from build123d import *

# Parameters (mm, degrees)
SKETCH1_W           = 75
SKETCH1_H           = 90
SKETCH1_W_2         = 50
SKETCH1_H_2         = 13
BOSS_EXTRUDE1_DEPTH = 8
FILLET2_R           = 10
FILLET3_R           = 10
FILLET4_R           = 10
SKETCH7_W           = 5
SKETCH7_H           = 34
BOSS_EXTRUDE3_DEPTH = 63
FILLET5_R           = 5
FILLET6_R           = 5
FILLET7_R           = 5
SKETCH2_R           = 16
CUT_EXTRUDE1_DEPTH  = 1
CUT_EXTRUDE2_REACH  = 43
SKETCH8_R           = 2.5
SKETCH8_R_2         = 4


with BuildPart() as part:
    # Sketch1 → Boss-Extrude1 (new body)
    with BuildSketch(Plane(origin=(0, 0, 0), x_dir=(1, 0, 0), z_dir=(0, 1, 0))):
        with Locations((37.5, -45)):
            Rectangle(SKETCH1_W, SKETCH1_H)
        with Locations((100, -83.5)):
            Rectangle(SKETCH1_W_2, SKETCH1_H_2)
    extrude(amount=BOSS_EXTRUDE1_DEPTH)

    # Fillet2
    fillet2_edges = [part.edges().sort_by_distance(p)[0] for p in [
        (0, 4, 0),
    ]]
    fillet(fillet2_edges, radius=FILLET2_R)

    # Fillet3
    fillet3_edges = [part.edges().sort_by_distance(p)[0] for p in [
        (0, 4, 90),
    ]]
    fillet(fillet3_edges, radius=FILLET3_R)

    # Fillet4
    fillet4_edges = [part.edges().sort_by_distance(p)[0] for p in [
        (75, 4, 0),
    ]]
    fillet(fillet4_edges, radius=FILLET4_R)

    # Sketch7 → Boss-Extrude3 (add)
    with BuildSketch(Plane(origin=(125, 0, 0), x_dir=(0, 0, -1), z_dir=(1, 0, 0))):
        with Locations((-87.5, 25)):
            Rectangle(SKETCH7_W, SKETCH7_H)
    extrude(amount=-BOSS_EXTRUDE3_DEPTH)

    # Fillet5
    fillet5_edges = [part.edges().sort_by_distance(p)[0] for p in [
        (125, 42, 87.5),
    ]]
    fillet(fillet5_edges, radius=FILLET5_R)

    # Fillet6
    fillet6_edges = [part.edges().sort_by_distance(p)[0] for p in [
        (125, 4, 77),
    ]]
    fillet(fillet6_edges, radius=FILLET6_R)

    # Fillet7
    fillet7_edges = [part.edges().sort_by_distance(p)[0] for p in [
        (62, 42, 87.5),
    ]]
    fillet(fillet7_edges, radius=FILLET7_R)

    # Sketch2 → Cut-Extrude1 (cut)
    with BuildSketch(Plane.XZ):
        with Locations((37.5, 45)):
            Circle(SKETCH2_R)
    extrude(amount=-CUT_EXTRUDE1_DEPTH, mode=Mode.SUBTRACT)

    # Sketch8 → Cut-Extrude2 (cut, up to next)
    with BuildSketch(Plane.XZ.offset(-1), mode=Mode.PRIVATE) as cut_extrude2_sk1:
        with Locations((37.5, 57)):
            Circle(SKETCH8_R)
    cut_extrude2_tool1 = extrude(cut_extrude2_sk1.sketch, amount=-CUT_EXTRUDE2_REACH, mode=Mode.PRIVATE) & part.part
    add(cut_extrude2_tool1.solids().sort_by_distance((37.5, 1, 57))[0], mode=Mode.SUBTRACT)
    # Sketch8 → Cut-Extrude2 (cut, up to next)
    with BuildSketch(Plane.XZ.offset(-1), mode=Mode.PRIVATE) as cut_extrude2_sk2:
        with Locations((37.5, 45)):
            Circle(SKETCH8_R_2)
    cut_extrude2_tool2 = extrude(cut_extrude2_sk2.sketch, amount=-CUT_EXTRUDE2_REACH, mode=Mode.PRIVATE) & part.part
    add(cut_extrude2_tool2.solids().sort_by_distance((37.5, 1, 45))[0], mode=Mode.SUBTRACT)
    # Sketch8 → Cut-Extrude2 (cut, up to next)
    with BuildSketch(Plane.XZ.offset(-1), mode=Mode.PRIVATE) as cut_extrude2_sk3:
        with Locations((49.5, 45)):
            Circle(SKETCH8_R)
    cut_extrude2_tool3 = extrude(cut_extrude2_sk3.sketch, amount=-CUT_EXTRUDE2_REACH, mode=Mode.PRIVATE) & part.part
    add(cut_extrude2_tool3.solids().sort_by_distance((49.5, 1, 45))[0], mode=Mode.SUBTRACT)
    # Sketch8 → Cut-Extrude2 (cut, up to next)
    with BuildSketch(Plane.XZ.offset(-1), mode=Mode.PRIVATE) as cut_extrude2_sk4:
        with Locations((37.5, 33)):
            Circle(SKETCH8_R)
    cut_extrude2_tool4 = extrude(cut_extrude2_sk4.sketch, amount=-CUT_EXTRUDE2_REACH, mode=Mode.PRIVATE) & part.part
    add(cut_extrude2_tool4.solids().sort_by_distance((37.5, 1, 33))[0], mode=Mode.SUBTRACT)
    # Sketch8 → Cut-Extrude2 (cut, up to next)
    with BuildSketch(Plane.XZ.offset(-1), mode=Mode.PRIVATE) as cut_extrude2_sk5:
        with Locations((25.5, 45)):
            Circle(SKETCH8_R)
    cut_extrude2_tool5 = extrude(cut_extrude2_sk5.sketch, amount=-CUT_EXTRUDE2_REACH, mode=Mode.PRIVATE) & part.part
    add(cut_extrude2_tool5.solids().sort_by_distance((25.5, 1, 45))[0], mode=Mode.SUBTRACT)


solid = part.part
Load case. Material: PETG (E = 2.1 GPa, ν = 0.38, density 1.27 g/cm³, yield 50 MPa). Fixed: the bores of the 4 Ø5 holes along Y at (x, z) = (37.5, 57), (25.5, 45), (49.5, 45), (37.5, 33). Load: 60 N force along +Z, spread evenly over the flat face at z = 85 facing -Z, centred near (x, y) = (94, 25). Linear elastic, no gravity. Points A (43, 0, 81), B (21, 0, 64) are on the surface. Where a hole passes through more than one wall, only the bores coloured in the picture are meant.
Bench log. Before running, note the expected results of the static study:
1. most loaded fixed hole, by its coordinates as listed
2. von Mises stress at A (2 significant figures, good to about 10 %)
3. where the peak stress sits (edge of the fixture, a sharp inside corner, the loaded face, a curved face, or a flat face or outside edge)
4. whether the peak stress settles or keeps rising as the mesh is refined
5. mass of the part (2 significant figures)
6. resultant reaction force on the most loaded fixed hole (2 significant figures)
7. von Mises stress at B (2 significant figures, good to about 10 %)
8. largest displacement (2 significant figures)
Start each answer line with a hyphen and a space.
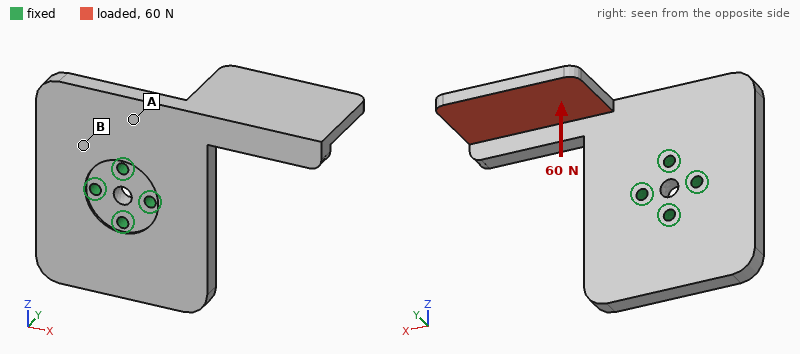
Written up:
- (49.5, 45)
- 2.2 MPa
- a sharp inside corner
- keeps rising
- 86 g
- 100 N
- 1.2 MPa
- 1.7 mm
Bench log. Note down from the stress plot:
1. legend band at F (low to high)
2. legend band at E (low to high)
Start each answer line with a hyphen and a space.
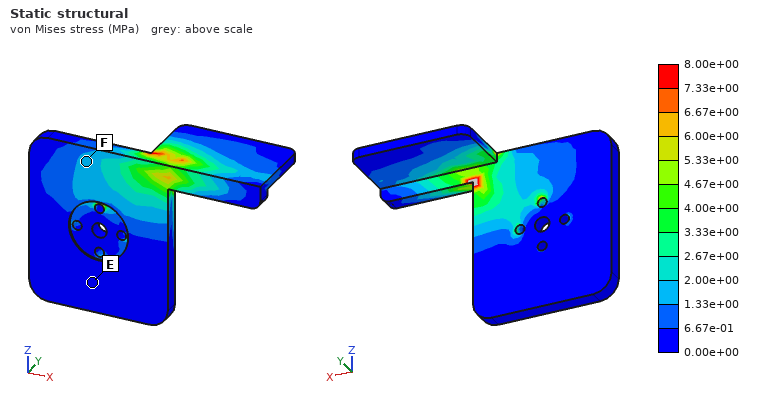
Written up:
- 1.33e+00 to 2.00e+00 MPa
- 0.00e+00 to 6.67e-01 MPa
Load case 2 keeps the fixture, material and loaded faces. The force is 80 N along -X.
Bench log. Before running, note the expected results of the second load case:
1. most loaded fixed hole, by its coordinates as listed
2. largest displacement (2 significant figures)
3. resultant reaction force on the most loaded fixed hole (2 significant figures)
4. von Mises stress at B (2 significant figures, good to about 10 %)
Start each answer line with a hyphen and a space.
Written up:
- (37.5, 57)
- 1.6 mm
- 100 N
- 0.59 MPa
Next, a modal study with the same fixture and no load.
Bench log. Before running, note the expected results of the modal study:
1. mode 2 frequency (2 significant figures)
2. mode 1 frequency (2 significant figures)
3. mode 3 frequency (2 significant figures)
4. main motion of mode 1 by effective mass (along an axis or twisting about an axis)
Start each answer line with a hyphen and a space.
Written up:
- 370 Hz
- 200 Hz
- 660 Hz
- along Y
